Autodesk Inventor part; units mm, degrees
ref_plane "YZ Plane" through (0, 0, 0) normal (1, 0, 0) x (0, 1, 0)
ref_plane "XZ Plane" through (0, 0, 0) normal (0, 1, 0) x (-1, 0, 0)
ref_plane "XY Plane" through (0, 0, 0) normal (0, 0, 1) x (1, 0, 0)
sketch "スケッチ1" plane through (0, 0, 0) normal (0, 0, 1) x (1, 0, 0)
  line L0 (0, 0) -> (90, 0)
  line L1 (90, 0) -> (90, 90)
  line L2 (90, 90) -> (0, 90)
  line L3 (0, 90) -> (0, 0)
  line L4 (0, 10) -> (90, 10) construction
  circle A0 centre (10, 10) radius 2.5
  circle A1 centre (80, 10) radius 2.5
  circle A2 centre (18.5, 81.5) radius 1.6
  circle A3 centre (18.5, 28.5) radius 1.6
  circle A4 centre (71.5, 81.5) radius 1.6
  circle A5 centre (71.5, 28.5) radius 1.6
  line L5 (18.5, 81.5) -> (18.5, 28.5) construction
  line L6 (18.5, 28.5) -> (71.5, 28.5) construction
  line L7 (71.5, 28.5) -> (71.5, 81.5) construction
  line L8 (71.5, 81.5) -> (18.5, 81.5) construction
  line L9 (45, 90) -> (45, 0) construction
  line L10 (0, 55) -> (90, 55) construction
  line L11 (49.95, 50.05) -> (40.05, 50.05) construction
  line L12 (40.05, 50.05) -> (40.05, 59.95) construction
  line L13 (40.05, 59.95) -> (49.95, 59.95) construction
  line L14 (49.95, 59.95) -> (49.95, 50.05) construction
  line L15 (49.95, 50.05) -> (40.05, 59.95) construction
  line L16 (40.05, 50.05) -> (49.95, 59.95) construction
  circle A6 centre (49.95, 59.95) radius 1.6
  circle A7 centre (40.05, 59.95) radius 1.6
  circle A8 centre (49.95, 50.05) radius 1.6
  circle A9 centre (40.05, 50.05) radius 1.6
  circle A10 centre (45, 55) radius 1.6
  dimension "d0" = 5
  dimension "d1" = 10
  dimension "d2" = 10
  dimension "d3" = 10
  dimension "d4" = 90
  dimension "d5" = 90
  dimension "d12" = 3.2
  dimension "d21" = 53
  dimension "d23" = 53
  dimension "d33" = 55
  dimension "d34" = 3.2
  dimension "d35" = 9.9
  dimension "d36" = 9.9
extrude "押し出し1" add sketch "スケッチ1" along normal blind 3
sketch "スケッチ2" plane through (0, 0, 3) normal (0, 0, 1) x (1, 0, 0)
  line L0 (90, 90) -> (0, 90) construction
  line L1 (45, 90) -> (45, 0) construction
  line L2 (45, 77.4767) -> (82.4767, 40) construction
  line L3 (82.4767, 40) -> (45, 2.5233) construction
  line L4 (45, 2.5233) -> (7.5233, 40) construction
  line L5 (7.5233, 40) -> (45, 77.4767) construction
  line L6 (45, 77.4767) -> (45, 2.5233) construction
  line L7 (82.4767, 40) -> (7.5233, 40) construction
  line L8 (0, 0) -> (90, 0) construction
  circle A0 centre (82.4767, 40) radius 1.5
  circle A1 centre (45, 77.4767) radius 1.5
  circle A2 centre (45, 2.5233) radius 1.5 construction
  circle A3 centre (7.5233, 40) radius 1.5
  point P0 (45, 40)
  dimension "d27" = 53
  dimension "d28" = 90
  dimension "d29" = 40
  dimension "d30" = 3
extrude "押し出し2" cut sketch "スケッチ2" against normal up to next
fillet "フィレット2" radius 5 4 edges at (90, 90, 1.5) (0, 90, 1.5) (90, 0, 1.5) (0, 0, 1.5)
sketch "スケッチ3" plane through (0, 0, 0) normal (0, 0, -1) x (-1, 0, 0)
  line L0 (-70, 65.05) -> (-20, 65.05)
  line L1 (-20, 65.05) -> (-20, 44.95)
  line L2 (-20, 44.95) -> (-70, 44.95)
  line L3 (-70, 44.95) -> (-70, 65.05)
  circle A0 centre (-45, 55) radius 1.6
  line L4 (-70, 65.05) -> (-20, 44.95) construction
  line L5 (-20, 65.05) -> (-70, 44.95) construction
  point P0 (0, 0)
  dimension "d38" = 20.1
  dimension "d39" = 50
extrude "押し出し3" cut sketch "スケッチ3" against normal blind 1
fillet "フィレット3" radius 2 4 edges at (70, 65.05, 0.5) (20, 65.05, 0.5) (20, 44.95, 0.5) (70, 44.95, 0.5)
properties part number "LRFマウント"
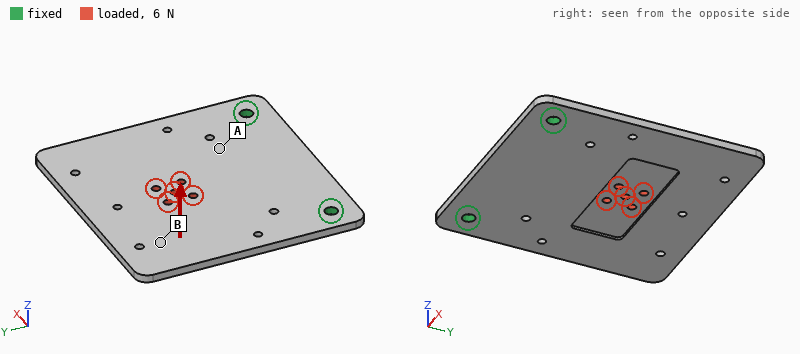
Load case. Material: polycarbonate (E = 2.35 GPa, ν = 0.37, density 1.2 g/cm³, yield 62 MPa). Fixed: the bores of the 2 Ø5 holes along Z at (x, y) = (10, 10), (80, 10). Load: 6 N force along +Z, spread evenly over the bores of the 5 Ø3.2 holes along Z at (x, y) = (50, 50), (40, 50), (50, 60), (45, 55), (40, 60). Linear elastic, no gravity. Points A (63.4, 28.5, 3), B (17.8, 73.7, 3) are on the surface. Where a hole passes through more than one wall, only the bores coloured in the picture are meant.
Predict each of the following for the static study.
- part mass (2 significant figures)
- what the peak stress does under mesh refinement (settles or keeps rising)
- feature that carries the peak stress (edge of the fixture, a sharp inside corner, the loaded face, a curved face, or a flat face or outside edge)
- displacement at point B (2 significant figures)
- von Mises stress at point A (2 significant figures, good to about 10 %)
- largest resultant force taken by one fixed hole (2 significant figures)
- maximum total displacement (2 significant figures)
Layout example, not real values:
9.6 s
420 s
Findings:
27 g
keeps rising
edge of the fixture
0.83 mm
1.1 MPa
3.0 N
1.2 mm
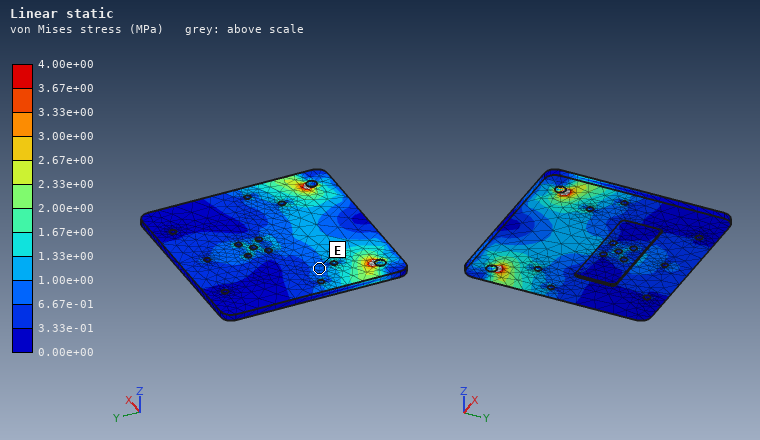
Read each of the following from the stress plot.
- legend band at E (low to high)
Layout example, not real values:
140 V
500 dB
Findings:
6.67e-01 to 1.00e+00 MPa
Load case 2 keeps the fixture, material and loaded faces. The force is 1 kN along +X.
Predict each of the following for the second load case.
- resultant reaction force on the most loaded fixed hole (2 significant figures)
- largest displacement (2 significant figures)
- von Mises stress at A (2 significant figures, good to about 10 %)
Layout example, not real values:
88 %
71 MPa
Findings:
800 N
0.68 mm
11 MPa
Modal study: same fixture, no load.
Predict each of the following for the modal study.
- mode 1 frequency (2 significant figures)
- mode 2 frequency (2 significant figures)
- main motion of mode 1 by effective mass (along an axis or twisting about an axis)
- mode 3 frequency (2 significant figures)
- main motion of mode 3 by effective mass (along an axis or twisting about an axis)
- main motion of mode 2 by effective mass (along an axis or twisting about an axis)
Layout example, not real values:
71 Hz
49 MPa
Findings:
95 Hz
230 Hz
along Z
550 Hz
along Z
twisting about Y
